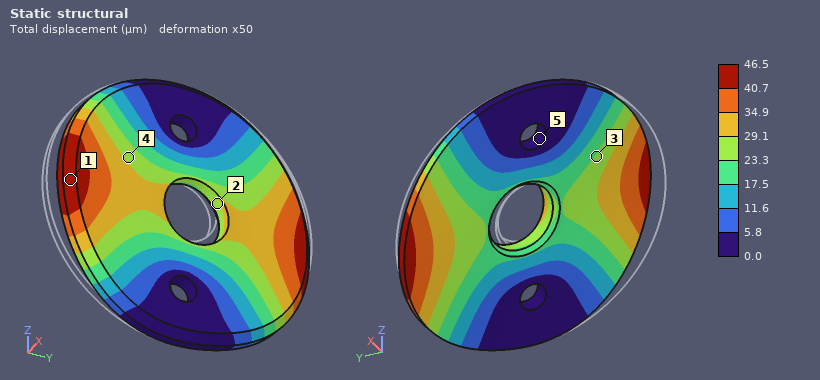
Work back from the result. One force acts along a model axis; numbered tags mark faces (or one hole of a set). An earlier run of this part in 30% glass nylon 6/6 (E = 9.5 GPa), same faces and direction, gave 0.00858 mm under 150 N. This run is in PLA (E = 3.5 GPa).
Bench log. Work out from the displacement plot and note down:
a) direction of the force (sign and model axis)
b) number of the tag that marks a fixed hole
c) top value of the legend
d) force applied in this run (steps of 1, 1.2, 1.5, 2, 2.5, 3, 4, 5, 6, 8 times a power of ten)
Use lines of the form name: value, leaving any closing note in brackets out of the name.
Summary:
direction of the force: +Y
number of the tag that marks a fixed hole: 5
top value of the legend: 46.5 µm
force applied in this run: 300 N
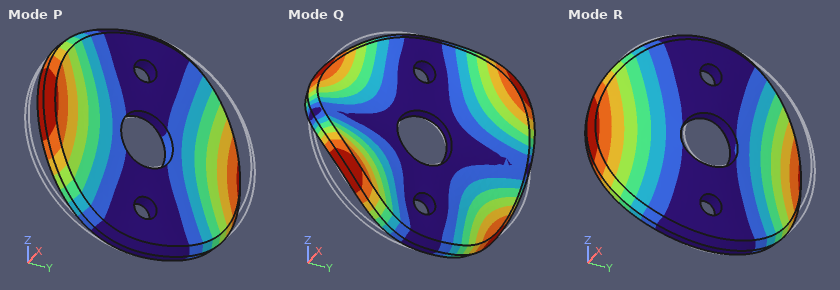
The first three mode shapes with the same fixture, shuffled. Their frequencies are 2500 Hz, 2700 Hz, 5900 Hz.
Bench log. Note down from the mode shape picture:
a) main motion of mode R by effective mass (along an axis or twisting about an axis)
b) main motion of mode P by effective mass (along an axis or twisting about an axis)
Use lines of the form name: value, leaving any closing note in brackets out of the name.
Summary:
main motion of mode R by effective mass: along X
main motion of mode P by effective mass: twisting about Z
